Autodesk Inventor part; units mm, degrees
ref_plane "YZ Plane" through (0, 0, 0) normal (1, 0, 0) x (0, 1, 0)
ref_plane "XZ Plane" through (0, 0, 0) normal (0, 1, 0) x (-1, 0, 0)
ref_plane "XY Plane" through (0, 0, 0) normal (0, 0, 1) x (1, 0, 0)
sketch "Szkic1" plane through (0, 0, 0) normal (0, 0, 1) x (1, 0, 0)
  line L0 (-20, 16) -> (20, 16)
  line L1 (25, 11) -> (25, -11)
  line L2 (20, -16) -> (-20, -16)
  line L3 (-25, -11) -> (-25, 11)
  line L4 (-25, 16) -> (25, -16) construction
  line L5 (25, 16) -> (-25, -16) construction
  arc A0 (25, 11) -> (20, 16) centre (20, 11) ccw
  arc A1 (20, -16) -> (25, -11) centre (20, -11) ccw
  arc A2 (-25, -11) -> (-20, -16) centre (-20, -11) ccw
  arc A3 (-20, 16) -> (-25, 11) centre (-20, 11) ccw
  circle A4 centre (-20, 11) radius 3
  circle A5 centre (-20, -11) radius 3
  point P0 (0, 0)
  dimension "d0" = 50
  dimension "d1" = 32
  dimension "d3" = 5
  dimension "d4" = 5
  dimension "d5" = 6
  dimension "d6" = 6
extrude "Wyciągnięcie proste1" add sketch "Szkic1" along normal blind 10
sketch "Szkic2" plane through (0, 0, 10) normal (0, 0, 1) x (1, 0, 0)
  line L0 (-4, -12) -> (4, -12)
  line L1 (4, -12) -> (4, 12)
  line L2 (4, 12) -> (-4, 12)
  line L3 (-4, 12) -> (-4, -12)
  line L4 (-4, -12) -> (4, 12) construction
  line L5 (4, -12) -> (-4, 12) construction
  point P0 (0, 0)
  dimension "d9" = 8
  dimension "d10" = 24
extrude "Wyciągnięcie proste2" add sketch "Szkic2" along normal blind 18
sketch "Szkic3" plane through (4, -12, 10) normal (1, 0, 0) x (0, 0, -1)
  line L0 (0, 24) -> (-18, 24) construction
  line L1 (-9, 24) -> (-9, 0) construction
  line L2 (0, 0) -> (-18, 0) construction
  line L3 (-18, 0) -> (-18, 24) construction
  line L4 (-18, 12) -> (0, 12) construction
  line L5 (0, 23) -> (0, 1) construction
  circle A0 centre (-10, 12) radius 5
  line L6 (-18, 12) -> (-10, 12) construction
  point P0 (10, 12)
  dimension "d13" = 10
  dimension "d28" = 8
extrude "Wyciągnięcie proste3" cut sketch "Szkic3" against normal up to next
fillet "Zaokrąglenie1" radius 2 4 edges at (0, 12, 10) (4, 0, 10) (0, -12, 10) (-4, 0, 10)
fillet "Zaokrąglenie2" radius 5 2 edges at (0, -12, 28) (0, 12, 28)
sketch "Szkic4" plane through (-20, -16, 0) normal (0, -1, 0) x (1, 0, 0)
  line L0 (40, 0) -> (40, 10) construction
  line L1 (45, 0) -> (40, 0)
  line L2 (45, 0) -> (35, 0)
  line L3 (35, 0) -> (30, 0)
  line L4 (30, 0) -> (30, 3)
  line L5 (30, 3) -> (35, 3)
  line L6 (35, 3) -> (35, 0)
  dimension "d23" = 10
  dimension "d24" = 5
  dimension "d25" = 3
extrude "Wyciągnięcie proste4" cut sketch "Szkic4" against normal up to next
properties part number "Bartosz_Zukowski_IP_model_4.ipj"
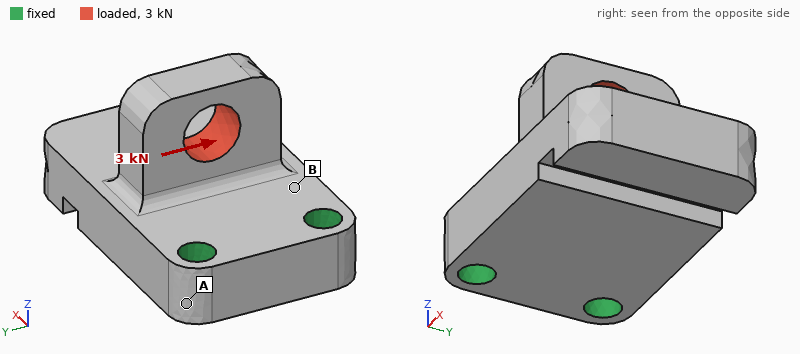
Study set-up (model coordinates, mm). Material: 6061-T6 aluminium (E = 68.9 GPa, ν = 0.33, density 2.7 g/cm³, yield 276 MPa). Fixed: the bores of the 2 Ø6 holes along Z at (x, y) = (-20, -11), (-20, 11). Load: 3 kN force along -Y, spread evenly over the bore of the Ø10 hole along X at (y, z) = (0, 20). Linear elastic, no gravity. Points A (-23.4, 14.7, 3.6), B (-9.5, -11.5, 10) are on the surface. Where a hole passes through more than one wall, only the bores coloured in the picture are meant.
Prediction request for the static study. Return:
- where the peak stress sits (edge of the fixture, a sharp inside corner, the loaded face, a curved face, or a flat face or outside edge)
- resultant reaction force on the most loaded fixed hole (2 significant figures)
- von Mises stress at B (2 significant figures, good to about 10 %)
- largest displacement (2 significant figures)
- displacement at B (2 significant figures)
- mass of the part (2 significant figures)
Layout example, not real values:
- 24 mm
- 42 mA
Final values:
- a curved face
- 3.2 kN
- 56 MPa
- 78 µm
- 14 µm
- 47 g
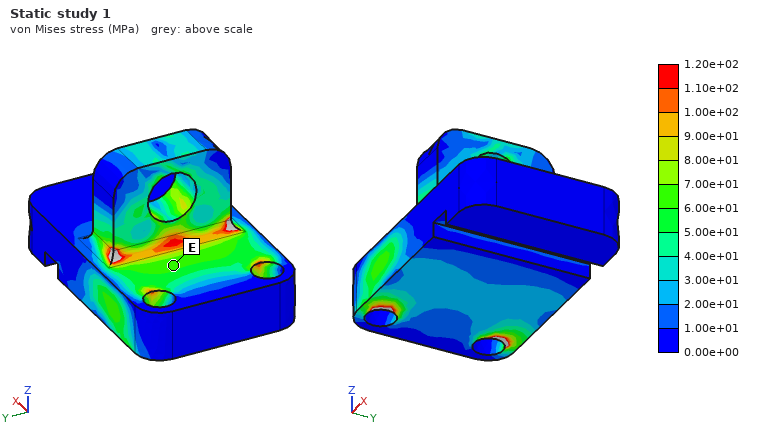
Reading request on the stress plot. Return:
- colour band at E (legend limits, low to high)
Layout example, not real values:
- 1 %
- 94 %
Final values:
- 6.00e+01 to 7.00e+01 MPa
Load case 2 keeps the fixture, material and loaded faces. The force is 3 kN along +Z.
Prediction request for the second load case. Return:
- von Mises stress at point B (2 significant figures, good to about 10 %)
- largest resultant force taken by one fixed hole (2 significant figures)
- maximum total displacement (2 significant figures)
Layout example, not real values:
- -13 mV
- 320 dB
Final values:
- 59 MPa
- 1.5 kN
- 0.13 mm
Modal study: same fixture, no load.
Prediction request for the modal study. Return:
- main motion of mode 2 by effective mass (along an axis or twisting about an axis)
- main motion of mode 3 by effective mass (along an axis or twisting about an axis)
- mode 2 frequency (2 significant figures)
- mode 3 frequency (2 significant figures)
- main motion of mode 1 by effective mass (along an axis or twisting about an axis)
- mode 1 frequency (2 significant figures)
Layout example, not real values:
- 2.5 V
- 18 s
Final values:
- along Y
- along Y
- 9700 Hz
- 10 kHz
- along Z
- 3900 Hz
